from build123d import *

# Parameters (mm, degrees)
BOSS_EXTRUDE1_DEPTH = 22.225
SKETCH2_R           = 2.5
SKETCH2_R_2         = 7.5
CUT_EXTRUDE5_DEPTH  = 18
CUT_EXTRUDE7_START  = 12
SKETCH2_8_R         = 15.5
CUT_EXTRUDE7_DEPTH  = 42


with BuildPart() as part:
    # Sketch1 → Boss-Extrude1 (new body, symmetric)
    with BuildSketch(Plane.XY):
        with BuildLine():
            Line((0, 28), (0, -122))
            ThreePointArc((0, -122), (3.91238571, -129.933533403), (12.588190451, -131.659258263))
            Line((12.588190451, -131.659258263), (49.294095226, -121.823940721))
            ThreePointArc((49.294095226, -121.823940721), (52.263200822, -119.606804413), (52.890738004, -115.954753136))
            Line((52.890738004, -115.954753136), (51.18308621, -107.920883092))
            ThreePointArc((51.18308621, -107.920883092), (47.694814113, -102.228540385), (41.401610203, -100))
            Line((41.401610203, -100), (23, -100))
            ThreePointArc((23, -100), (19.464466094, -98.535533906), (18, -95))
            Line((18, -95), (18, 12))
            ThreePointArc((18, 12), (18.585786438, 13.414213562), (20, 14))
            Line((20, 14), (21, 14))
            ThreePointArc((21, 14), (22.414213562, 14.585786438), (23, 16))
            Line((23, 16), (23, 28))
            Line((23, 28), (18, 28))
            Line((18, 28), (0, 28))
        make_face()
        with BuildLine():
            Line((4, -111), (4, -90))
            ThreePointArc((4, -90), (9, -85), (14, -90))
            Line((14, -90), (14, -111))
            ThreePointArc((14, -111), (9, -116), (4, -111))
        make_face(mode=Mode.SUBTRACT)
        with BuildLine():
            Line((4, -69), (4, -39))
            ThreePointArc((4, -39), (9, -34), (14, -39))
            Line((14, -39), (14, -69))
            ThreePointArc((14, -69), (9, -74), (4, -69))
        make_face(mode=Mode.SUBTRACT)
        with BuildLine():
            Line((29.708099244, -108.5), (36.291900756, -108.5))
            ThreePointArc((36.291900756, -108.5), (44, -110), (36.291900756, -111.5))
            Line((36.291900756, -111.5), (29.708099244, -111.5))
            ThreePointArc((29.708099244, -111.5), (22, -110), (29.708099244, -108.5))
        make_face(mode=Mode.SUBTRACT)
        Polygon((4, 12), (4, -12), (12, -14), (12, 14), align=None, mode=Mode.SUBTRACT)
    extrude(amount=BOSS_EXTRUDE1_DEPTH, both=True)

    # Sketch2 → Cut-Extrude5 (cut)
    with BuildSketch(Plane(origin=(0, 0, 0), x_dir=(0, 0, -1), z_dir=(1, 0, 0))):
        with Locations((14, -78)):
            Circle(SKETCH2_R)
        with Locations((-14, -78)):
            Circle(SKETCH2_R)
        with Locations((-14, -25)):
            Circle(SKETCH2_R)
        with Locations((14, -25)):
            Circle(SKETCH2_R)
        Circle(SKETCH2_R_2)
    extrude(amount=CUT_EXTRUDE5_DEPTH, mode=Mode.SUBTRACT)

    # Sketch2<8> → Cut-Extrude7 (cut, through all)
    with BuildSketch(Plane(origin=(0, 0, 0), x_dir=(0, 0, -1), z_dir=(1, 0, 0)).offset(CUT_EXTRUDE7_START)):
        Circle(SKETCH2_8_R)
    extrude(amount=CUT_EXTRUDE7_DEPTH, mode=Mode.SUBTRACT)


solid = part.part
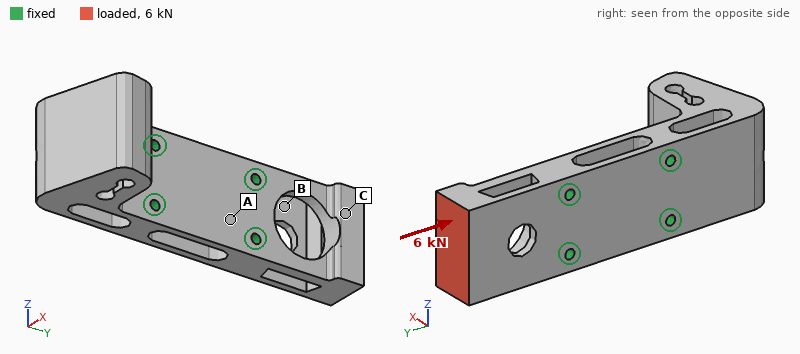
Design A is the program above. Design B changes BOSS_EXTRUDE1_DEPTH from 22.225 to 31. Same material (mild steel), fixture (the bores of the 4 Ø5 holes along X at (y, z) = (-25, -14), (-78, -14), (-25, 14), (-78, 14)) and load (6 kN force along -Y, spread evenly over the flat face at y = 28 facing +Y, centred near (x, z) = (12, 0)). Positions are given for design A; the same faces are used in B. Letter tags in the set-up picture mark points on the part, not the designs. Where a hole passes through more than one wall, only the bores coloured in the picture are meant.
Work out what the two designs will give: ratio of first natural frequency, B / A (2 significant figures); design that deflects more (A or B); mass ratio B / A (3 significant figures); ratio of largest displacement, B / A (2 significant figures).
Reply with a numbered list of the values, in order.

1. 0.98
2. A
3. 1.42
4. 0.54
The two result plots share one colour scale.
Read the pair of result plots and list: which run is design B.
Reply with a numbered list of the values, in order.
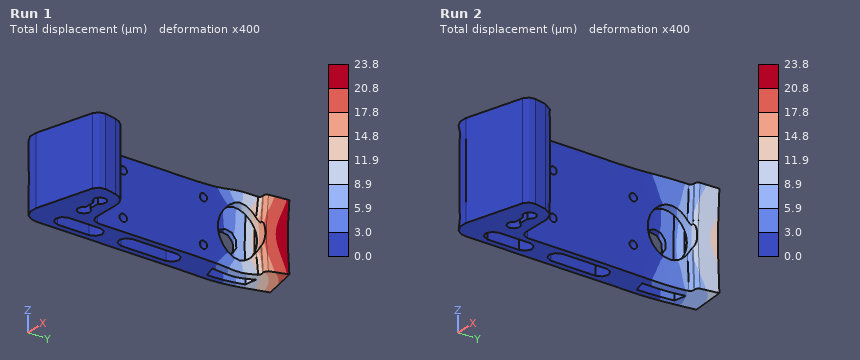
1. Run 2
